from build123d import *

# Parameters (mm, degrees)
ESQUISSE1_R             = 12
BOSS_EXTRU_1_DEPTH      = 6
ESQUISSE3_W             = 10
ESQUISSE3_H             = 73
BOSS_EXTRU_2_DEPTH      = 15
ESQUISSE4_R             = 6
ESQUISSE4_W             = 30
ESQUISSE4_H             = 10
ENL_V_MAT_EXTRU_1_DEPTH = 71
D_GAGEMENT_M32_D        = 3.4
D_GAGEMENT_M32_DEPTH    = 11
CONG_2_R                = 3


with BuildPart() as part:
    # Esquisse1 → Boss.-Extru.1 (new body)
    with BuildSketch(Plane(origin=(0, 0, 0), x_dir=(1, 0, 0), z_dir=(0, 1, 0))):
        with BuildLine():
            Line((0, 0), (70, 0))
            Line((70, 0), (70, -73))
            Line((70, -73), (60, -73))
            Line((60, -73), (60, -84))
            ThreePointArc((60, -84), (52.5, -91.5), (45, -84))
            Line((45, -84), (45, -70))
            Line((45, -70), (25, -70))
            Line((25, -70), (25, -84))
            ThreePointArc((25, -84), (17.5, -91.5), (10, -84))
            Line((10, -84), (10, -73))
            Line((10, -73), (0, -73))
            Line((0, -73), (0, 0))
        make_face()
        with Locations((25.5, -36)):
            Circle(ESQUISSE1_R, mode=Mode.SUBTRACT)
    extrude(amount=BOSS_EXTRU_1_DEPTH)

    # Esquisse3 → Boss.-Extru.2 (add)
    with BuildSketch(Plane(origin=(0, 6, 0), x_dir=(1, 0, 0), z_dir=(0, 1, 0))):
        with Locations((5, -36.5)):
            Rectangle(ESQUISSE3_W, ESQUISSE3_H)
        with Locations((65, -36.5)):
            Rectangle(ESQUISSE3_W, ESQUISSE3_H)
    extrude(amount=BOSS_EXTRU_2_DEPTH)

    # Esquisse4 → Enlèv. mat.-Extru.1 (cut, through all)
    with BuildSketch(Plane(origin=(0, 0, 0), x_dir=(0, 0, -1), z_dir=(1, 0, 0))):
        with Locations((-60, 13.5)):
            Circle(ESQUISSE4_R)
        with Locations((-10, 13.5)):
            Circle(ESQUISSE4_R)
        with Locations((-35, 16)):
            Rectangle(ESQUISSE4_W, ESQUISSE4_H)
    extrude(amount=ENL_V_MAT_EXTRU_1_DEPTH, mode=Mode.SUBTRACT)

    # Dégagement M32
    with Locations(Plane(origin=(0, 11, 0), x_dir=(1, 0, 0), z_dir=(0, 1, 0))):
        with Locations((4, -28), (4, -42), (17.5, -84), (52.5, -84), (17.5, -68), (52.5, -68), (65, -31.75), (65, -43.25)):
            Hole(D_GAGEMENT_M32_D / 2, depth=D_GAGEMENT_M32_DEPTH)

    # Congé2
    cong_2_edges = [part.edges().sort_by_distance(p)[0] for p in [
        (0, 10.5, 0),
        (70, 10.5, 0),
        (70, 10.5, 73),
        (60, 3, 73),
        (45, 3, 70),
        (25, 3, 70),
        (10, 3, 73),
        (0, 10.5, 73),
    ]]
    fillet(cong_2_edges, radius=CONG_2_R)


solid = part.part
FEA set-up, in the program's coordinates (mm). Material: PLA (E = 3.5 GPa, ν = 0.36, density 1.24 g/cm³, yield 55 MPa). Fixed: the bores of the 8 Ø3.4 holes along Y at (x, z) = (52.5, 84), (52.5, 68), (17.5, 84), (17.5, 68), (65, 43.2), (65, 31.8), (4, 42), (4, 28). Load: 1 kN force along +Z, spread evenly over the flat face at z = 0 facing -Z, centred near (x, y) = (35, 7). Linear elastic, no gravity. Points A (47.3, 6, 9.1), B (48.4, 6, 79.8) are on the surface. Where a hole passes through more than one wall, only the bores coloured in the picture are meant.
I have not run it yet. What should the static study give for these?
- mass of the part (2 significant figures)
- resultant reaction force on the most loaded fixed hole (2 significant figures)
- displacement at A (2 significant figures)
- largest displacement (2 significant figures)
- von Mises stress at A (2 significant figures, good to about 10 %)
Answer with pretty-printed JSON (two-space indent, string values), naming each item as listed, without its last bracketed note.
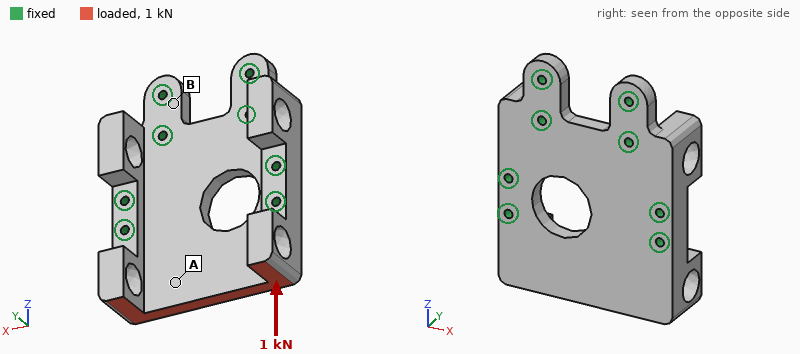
{
  "mass of the part": "51 g",
  "resultant reaction force on the most loaded fixed hole": "380 N",
  "displacement at A": "0.055 mm",
  "largest displacement": "0.18 mm",
  "von Mises stress at A": "2.4 MPa"
}
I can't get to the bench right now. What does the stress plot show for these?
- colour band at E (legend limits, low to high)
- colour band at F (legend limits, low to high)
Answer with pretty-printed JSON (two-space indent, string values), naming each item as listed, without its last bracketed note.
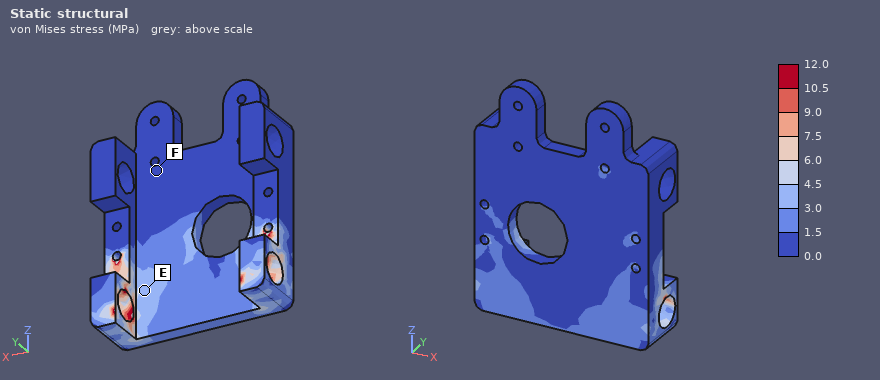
{
  "colour band at E": "3.0 to 4.5 MPa",
  "colour band at F": "0.0 to 1.5 MPa"
}
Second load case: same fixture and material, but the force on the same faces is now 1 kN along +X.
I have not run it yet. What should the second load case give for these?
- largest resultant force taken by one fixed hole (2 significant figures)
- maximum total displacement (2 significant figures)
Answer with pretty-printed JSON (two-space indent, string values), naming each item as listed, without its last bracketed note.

{
  "largest resultant force taken by one fixed hole": "650 N",
  "maximum total displacement": "0.36 mm"
}
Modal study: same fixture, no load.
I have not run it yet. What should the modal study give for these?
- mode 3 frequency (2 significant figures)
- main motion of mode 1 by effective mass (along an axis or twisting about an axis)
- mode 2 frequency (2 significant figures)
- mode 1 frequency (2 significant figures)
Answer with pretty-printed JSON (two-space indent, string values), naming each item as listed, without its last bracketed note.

{
  "mode 3 frequency": "3000 Hz",
  "main motion of mode 1 by effective mass": "along Y",
  "mode 2 frequency": "2500 Hz",
  "mode 1 frequency": "1700 Hz"
}
